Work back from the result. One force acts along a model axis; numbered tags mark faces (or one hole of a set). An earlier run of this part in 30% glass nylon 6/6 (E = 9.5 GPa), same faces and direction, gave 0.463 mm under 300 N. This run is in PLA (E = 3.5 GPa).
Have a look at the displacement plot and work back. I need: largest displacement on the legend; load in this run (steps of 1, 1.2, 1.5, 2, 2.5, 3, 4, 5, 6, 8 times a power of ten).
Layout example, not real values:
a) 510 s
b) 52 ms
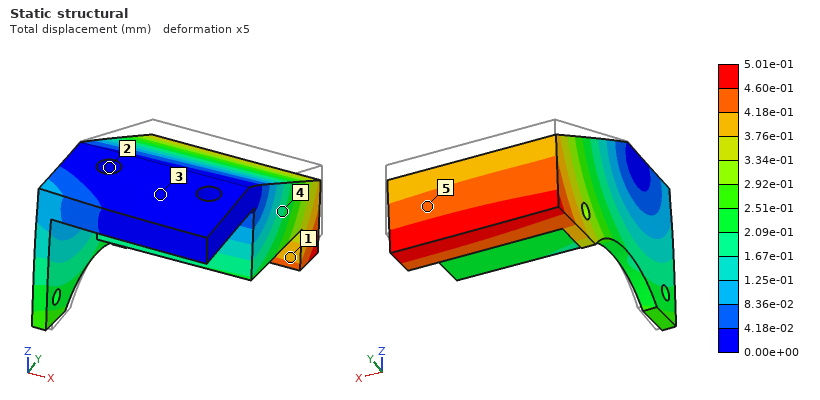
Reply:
a) 5.01e-01 mm
b) 120 N
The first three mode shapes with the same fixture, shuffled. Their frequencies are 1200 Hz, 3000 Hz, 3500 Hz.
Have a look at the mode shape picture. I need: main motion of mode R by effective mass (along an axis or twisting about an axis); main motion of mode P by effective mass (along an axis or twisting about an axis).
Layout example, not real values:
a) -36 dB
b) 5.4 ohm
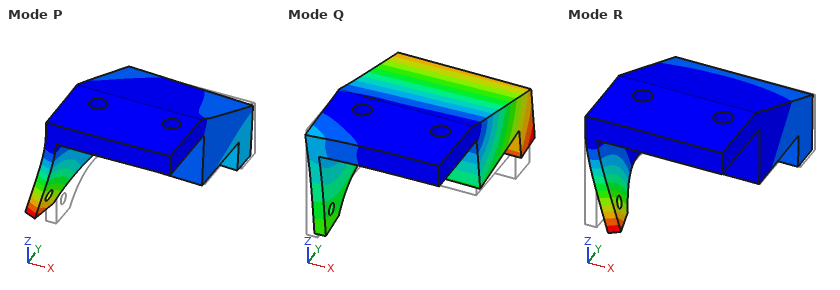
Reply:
a) along X
b) along X
